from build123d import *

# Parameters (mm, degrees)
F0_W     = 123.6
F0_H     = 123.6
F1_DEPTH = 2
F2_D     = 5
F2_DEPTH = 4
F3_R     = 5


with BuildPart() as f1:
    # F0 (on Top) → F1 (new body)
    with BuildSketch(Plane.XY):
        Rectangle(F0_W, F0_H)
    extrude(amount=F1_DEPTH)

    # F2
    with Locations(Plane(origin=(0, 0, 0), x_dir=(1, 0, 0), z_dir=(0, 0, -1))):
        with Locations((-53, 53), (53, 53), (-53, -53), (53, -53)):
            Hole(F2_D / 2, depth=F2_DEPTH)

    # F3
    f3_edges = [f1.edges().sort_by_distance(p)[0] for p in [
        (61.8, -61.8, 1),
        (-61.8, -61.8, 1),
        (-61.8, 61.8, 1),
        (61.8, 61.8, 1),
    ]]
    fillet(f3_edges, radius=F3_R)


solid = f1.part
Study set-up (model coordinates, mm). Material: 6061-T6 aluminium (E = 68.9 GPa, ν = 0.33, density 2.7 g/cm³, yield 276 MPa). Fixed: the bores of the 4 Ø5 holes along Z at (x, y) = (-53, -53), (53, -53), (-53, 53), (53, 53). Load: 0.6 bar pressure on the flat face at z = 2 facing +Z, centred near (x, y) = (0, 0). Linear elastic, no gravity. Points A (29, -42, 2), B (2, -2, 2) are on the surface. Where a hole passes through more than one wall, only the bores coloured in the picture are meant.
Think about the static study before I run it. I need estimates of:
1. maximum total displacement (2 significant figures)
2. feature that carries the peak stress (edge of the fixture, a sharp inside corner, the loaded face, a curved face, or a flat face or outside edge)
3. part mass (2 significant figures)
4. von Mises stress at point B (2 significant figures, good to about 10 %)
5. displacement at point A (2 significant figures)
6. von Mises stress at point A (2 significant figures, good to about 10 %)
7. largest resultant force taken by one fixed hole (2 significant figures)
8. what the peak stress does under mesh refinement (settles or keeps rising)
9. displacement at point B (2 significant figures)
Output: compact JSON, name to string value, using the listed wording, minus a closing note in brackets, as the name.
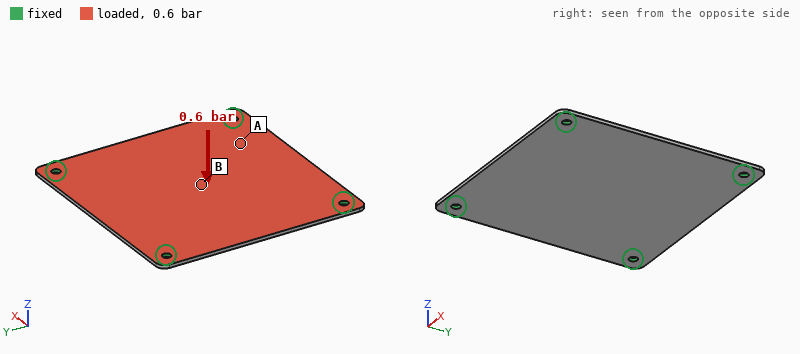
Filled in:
{"maximum total displacement": "1.1 mm", "feature that carries the peak stress": "edge of the fixture", "part mass": "82 g", "von Mises stress at point B": "56 MPa", "displacement at point A": "0.46 mm", "von Mises stress at point A": "23 MPa", "largest resultant force taken by one fixed hole": "230 N", "what the peak stress does under mesh refinement": "keeps rising", "displacement at point B": "1.1 mm"}
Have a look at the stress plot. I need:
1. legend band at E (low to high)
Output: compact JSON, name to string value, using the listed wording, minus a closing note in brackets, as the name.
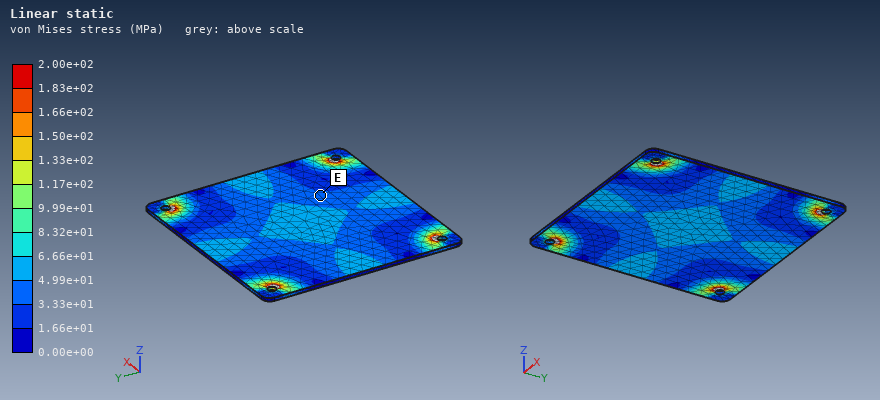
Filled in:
{"legend band at E": "3.33e+01 to 4.99e+01 MPa"}
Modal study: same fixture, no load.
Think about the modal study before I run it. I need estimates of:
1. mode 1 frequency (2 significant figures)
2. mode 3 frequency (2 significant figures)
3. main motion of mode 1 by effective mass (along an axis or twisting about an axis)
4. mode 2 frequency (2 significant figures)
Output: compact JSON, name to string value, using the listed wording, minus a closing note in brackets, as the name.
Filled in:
{"mode 1 frequency": "610 Hz", "mode 3 frequency": "1000 Hz", "main motion of mode 1 by effective mass": "along Z", "mode 2 frequency": "1000 Hz"}
